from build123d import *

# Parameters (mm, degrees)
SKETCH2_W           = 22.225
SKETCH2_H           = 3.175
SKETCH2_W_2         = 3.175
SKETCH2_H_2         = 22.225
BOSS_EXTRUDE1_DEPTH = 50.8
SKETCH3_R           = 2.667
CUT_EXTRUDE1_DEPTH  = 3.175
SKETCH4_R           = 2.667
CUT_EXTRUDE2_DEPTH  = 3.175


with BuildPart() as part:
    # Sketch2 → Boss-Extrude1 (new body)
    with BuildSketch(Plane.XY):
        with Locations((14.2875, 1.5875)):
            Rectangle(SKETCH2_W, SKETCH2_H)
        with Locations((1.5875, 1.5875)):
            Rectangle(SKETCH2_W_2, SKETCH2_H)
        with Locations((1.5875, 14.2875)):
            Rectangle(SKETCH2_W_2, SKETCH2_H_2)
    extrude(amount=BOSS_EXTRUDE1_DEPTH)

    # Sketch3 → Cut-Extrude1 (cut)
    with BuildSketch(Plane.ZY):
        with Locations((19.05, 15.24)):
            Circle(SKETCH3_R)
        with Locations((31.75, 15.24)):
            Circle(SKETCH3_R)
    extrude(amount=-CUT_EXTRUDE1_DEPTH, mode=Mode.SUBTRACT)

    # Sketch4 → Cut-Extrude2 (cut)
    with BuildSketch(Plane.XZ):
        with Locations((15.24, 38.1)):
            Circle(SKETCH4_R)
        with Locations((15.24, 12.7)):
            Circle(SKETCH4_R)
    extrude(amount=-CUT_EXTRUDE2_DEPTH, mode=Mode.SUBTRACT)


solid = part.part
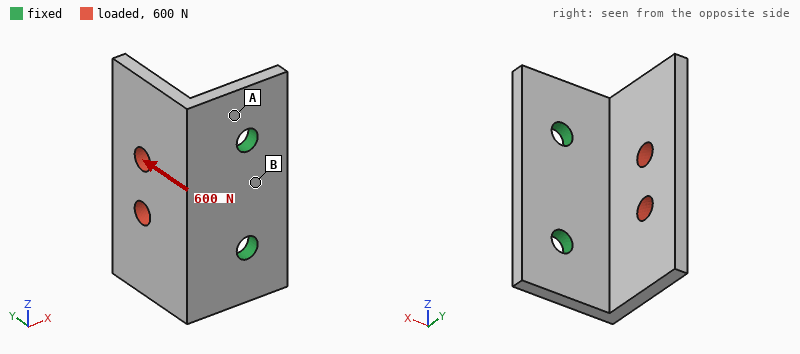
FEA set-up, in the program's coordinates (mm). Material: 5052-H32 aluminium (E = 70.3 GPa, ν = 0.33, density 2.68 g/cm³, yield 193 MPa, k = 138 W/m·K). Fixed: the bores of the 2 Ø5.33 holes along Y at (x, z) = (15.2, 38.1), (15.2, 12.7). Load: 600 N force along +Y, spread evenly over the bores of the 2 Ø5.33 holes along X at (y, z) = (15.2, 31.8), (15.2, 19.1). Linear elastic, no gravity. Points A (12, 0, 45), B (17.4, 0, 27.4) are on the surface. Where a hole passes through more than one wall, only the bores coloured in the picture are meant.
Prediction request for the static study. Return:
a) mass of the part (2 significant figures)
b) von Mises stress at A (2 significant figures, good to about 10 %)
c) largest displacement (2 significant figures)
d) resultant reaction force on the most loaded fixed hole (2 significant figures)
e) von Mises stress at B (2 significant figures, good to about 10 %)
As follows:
20 g
47 MPa
0.14 mm
300 N
17 MPa
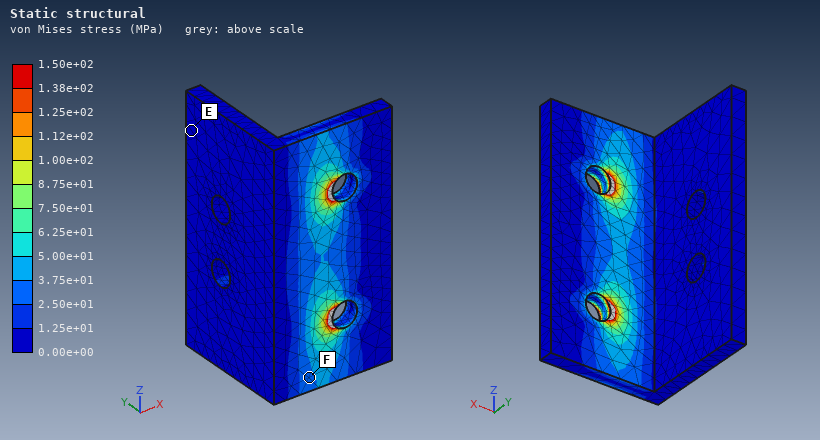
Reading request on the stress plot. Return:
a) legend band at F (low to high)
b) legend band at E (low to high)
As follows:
2.50e+01 to 3.75e+01 MPa
0.00e+00 to 1.25e+01 MPa
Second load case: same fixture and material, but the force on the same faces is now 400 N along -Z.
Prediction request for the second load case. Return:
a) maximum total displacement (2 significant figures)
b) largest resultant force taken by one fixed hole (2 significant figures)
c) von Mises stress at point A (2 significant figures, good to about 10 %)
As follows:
52 µm
320 N
22 MPa
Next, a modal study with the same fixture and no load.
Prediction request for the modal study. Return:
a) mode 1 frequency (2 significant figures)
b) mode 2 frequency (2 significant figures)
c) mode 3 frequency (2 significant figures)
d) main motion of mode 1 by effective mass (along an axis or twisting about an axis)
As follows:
2600 Hz
4200 Hz
6900 Hz
along X
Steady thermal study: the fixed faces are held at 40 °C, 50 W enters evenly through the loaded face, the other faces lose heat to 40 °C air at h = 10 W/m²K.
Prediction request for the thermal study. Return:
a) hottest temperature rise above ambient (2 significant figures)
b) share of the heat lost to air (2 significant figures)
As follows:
76 K
3.3 %
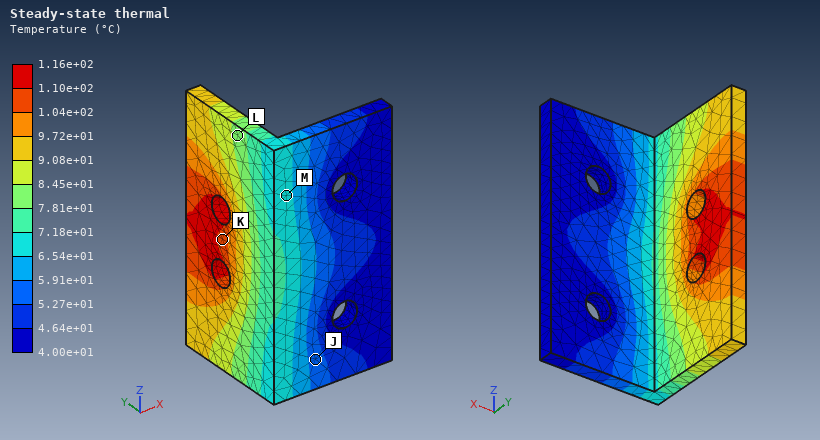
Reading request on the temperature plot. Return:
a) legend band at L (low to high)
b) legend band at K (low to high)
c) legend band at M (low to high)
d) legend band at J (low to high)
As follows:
7.81e+01 to 8.45e+01 °C
1.04e+02 to 1.10e+02 °C
6.54e+01 to 7.18e+01 °C
5.27e+01 to 5.91e+01 °C
